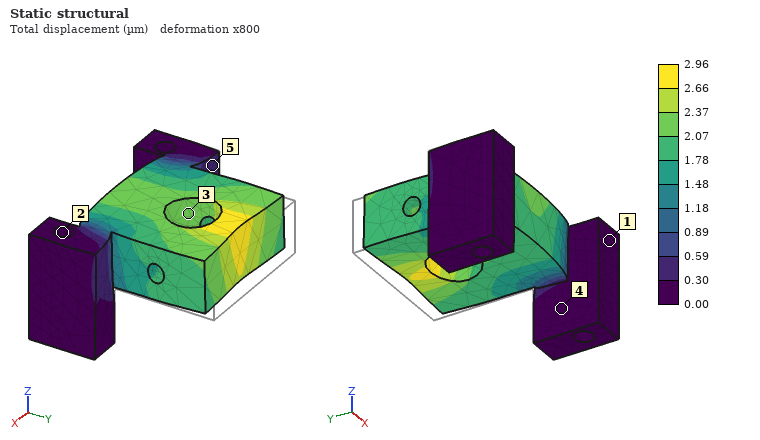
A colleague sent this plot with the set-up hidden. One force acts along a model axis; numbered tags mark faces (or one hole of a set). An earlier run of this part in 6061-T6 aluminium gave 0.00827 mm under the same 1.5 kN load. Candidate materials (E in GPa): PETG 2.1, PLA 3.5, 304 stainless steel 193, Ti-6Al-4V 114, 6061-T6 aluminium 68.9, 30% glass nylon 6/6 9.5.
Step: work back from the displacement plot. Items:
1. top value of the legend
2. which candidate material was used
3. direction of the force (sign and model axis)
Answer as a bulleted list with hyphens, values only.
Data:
- 2.96 µm
- 304 stainless steel
- -Y
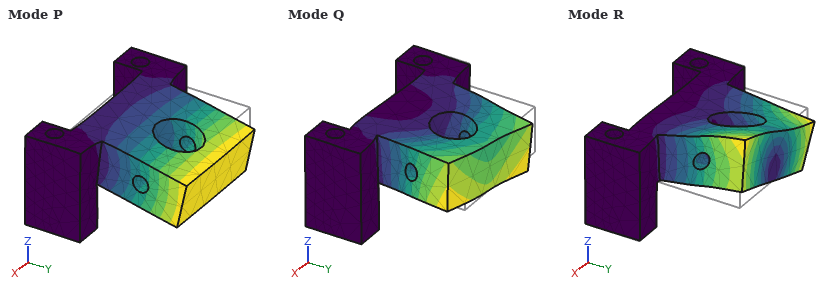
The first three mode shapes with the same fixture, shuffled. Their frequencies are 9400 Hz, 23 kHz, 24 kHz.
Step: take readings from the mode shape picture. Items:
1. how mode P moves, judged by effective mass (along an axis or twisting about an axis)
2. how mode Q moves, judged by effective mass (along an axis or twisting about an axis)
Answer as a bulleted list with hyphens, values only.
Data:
- along Z
- along X
